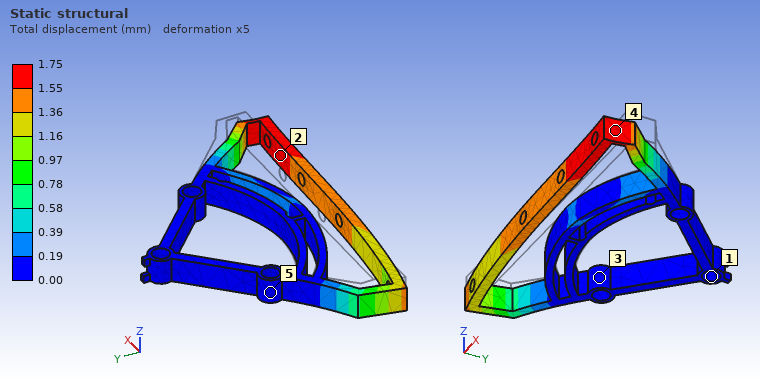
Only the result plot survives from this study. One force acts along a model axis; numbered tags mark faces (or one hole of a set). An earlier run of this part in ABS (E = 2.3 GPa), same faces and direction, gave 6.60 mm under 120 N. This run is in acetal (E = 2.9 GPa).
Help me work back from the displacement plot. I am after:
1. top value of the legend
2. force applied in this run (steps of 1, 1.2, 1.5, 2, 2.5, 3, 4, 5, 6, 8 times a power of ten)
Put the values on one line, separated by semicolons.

1.75 mm; 40 N
